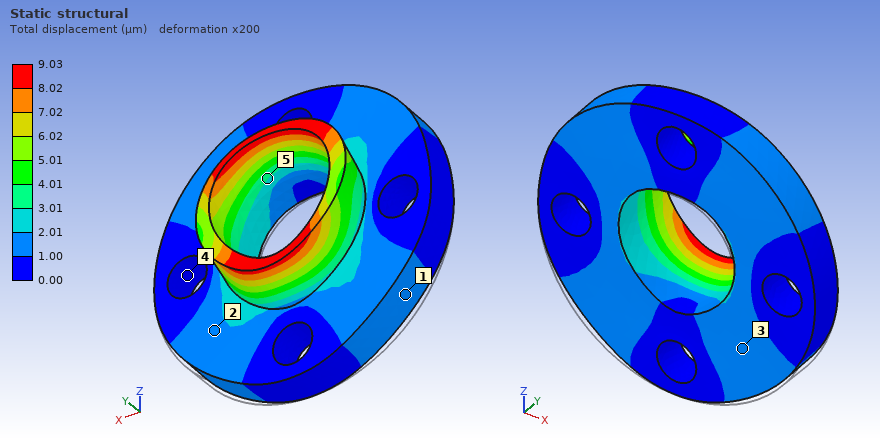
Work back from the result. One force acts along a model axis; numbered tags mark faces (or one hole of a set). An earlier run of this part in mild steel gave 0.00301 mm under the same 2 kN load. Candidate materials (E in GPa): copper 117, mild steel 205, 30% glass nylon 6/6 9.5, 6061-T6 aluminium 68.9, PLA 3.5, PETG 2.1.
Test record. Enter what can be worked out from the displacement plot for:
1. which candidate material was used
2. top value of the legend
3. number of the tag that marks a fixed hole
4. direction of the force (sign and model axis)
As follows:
6061-T6 aluminium
9.03 µm
4
+Z
